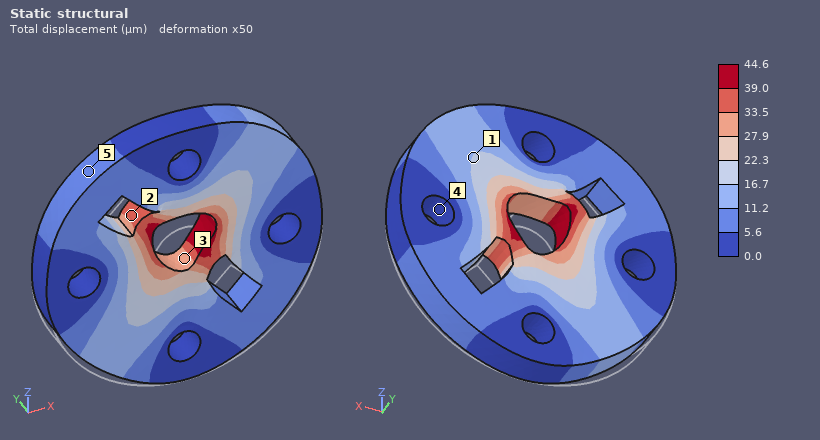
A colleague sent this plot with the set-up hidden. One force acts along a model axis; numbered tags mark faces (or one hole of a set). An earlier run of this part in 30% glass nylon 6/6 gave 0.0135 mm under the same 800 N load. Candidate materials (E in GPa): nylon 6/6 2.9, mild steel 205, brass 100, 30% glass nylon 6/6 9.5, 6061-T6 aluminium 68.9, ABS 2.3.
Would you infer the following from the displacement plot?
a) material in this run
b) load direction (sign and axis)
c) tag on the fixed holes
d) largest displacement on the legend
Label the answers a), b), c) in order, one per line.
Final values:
a) nylon 6/6
b) +Z
c) 4
d) 44.6 µm
